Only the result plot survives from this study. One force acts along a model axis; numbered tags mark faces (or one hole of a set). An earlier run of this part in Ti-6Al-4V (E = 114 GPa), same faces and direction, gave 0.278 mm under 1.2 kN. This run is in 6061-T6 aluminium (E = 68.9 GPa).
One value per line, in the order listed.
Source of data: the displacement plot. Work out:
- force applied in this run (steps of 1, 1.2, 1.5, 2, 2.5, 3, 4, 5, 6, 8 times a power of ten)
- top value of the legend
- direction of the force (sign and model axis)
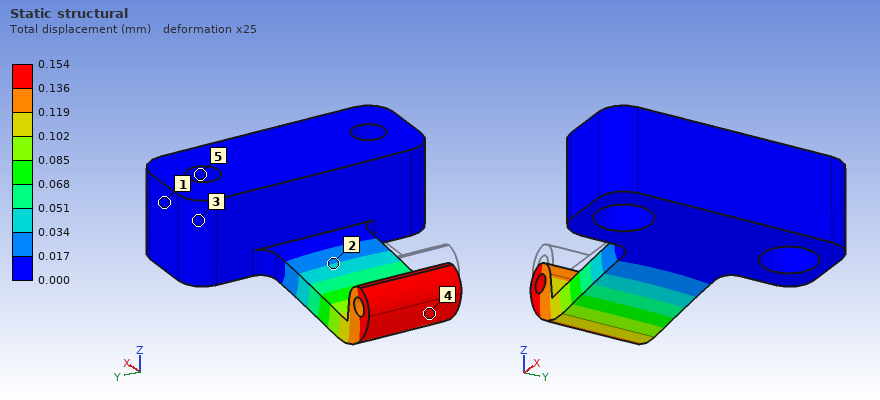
400 N
0.154 mm
-Z
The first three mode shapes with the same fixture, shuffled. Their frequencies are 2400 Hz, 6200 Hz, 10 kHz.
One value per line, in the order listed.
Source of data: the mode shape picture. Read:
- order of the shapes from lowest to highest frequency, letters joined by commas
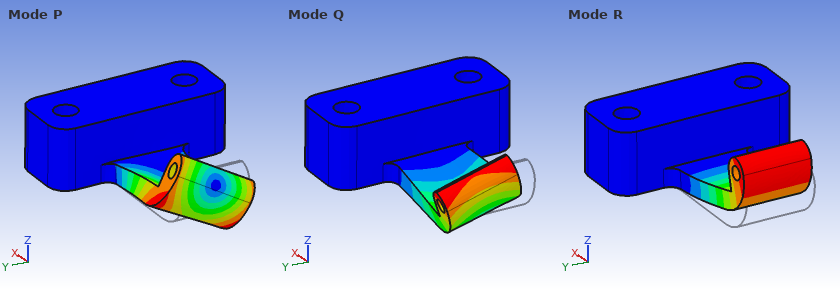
R, Q, P
